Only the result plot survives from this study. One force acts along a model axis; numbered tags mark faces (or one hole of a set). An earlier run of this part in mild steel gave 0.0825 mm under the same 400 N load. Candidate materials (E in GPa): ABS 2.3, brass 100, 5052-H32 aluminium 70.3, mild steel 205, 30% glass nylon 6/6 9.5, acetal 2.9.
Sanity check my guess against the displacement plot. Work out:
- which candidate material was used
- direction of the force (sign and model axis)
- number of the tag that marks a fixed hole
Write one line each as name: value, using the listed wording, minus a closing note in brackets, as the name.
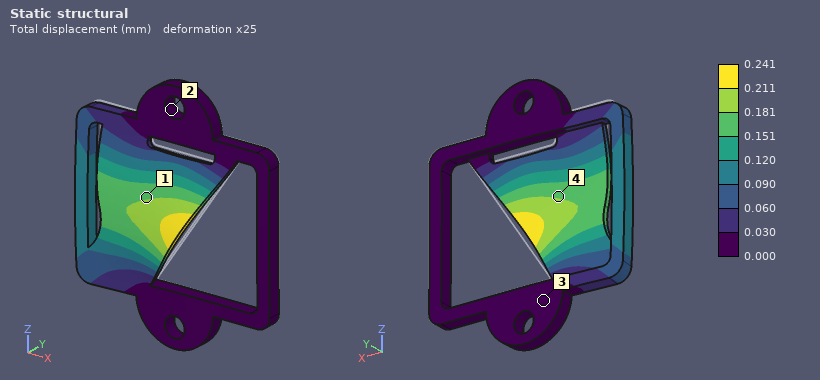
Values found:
which candidate material was used: 5052-H32 aluminium
direction of the force: -Y
number of the tag that marks a fixed hole: 2
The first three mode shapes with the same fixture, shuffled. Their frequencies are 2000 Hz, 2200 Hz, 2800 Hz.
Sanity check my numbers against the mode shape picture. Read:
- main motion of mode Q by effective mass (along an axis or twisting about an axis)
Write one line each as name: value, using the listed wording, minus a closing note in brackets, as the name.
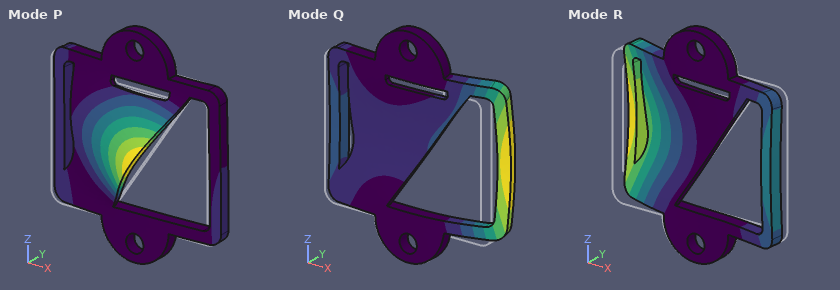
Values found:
main motion of mode Q by effective mass: along Y
